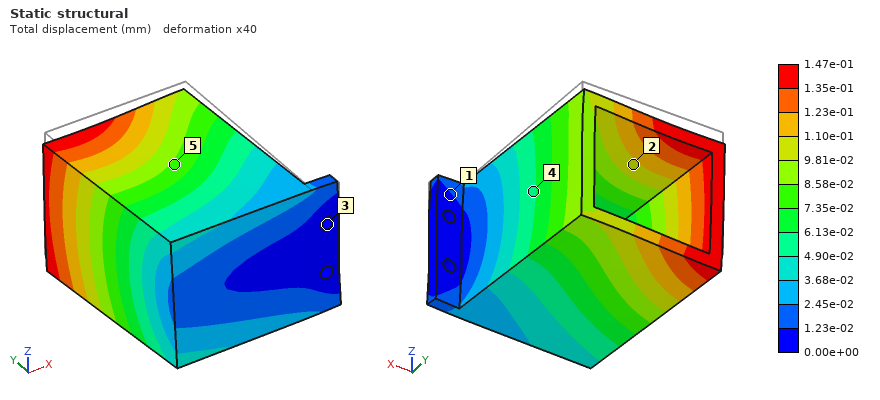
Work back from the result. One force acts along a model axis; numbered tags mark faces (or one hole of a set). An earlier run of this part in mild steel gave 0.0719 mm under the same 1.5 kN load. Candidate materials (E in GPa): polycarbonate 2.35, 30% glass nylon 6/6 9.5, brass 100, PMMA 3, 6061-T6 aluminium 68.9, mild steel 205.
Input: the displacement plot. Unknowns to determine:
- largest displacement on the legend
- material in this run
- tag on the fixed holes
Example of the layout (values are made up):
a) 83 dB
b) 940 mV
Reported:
a) 1.47e-01 mm
b) brass
c) 3
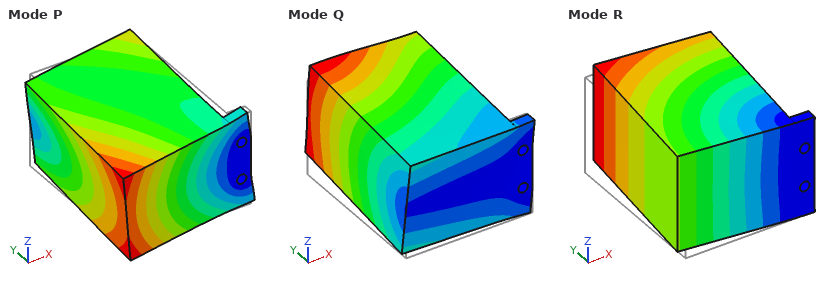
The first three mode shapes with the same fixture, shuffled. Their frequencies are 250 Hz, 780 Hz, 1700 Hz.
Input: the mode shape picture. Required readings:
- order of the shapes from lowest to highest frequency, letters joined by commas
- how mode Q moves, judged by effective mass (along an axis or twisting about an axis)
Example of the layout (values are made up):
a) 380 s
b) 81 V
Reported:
a) R, Q, P
b) along Z
